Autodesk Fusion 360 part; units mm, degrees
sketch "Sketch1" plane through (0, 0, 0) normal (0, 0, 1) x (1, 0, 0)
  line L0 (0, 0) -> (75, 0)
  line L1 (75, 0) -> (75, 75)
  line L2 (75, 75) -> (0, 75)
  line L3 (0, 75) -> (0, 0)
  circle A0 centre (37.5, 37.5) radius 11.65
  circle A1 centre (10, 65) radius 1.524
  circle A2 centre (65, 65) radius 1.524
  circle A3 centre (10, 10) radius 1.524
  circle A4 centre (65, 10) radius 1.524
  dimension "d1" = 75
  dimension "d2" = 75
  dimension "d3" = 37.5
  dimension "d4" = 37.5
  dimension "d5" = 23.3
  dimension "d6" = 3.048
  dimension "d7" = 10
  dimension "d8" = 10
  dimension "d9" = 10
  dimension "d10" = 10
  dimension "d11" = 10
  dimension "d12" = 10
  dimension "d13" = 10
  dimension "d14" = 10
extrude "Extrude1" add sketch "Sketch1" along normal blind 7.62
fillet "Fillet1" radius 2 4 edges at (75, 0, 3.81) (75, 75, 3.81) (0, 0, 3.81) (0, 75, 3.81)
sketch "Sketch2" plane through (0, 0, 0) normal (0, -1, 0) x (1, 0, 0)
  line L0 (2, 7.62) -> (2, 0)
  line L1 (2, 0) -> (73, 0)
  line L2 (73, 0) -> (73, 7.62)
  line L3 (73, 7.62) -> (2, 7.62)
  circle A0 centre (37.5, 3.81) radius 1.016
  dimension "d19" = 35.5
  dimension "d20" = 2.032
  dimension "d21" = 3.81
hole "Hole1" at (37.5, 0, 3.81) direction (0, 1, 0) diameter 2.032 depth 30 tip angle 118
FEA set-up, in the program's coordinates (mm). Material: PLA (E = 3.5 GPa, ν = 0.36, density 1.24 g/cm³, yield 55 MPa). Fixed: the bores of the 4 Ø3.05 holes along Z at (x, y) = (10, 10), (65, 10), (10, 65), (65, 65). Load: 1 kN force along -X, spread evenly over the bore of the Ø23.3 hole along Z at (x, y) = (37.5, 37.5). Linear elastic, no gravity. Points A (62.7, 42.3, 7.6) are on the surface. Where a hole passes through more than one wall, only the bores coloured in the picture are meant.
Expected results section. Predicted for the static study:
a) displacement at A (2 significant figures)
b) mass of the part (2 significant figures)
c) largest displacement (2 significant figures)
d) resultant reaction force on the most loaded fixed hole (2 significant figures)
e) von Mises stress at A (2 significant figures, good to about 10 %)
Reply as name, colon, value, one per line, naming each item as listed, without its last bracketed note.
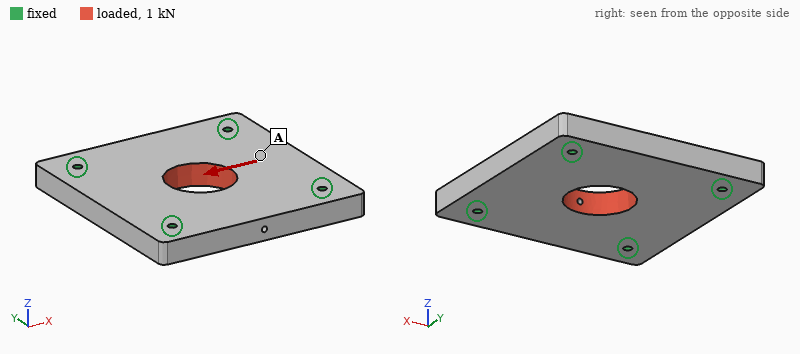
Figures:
displacement at A: 20 µm
mass of the part: 49 g
largest displacement: 26 µm
resultant reaction force on the most loaded fixed hole: 270 N
von Mises stress at A: 0.87 MPa
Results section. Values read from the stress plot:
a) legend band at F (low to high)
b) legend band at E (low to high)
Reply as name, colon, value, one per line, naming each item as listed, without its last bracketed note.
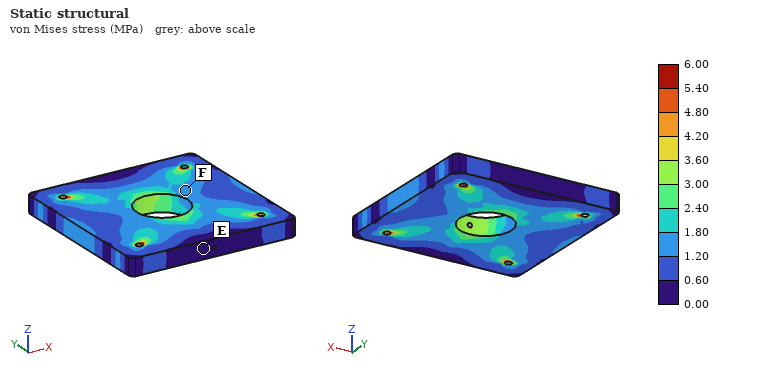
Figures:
legend band at F: 1.20 to 1.80 MPa
legend band at E: 0.00 to 0.60 MPa
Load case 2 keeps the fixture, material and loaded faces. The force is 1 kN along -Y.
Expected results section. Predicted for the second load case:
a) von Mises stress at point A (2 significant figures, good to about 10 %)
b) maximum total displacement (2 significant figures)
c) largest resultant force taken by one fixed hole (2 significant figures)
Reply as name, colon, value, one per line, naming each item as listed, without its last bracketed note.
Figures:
von Mises stress at point A: 1.1 MPa
maximum total displacement: 26 µm
largest resultant force taken by one fixed hole: 270 N
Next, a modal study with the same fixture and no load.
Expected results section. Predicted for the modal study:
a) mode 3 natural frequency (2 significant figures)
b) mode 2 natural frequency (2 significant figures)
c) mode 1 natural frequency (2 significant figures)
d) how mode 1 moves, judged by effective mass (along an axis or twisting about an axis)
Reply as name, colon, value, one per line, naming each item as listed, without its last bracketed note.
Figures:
mode 3 natural frequency: 3700 Hz
mode 2 natural frequency: 3600 Hz
mode 1 natural frequency: 2600 Hz
how mode 1 moves, judged by effective mass: along Z
